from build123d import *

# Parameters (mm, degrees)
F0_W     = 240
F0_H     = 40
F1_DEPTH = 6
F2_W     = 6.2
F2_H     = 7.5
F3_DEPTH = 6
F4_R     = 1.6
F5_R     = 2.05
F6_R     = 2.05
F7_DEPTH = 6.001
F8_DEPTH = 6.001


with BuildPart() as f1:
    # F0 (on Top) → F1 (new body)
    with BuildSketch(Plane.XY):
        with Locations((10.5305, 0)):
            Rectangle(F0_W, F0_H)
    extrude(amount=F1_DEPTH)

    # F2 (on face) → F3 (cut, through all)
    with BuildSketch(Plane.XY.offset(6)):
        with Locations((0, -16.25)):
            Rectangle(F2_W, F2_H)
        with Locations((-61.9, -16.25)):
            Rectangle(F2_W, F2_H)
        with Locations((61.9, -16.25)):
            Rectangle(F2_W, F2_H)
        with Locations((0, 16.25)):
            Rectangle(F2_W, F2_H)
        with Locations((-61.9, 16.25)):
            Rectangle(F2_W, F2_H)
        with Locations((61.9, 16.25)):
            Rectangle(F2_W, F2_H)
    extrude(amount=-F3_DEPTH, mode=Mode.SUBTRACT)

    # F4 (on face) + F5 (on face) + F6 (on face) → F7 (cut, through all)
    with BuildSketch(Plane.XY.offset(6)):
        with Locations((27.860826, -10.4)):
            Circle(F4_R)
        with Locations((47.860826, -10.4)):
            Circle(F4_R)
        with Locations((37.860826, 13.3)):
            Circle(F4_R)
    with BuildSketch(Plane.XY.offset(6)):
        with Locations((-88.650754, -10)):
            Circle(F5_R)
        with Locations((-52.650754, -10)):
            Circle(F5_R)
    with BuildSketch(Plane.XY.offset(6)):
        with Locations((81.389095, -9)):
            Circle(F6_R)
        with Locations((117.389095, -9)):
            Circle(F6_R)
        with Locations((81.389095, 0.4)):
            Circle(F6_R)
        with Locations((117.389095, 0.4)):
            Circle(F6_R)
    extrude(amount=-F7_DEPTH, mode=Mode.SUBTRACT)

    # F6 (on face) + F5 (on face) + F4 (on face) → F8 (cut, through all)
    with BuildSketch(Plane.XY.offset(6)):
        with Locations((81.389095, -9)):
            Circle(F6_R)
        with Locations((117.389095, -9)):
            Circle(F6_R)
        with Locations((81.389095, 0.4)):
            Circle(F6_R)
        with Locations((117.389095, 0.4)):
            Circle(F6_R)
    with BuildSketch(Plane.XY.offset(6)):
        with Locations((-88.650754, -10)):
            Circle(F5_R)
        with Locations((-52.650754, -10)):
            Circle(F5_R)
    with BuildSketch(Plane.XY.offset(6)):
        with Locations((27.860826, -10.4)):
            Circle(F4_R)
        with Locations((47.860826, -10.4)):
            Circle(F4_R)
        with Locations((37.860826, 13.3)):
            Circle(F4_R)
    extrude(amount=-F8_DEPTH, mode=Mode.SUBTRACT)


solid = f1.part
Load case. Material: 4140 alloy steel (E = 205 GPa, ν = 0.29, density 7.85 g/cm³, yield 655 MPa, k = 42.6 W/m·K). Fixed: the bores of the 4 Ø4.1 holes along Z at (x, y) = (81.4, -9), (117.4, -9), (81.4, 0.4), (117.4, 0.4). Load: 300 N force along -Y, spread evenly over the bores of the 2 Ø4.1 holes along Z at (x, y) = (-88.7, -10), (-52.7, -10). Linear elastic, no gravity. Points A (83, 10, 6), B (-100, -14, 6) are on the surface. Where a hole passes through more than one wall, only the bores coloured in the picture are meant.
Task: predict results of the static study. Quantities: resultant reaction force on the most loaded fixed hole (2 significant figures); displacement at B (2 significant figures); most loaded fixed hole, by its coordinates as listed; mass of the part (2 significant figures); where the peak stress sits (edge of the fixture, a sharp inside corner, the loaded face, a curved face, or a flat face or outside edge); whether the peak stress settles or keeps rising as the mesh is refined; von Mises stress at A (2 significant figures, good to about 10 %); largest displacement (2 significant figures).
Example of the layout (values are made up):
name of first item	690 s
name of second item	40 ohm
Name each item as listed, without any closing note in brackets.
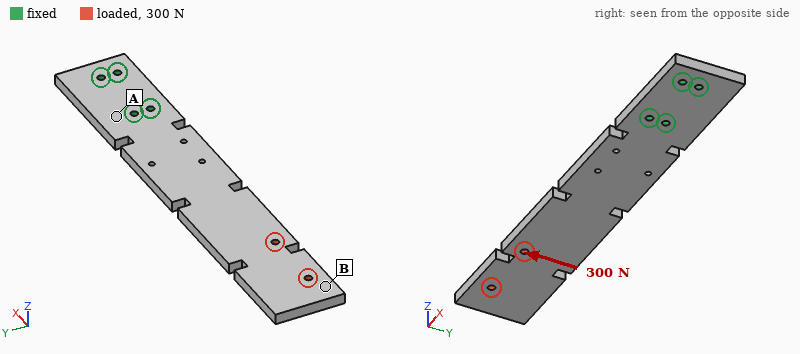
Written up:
resultant reaction force on the most loaded fixed hole	1.8 kN
displacement at B	0.16 mm
most loaded fixed hole, by its coordinates as listed	(81.4, -9)
mass of the part	430 g
where the peak stress sits	edge of the fixture
whether the peak stress settles or keeps rising as the mesh is refined	keeps rising
von Mises stress at A	16 MPa
largest displacement	0.18 mm
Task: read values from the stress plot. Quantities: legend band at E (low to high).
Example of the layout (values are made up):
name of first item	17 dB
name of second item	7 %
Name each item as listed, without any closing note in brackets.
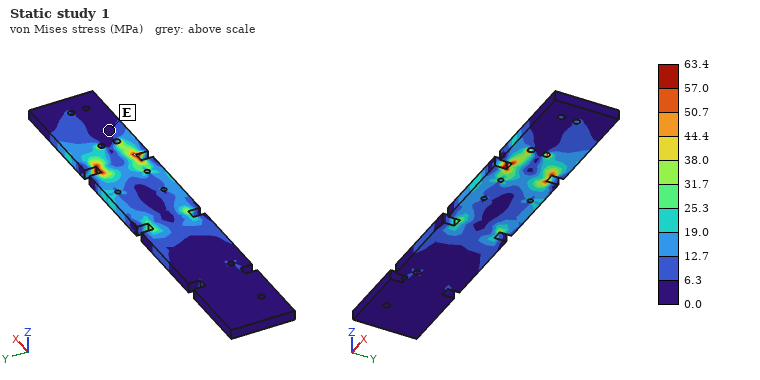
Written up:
legend band at E	0.0 to 6.3 MPa
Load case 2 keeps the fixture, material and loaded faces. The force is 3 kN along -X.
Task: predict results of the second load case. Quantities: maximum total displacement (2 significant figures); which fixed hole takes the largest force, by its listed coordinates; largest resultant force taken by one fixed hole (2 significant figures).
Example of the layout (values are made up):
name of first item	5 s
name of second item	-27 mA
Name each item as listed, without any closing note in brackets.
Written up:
maximum total displacement	0.17 mm
which fixed hole takes the largest force, by its listed coordinates	(81.4, -9)
largest resultant force taken by one fixed hole	2.2 kN
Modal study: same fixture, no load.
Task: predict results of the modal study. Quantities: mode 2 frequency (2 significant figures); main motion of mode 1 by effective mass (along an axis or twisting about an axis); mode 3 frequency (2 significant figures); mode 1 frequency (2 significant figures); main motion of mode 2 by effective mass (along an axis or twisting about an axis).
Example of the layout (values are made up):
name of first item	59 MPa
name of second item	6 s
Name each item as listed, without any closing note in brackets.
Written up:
mode 2 frequency	590 Hz
main motion of mode 1 by effective mass	along Z
mode 3 frequency	790 Hz
mode 1 frequency	130 Hz
main motion of mode 2 by effective mass	along Y
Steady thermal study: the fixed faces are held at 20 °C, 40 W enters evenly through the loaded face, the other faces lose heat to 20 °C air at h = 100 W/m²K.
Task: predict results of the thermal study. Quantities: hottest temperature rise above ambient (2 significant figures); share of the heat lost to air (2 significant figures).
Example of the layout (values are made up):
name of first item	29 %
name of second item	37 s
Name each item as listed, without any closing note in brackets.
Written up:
hottest temperature rise above ambient	76 K
share of the heat lost to air	99 %
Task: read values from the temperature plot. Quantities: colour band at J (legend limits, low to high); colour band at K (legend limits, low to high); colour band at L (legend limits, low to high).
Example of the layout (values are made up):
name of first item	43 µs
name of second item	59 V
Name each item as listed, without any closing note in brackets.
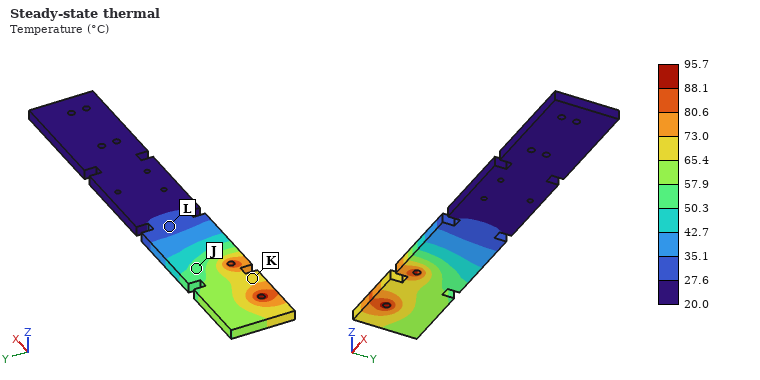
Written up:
colour band at J	50.3 to 57.9 °C
colour band at K	65.4 to 73.0 °C
colour band at L	27.6 to 35.1 °C
